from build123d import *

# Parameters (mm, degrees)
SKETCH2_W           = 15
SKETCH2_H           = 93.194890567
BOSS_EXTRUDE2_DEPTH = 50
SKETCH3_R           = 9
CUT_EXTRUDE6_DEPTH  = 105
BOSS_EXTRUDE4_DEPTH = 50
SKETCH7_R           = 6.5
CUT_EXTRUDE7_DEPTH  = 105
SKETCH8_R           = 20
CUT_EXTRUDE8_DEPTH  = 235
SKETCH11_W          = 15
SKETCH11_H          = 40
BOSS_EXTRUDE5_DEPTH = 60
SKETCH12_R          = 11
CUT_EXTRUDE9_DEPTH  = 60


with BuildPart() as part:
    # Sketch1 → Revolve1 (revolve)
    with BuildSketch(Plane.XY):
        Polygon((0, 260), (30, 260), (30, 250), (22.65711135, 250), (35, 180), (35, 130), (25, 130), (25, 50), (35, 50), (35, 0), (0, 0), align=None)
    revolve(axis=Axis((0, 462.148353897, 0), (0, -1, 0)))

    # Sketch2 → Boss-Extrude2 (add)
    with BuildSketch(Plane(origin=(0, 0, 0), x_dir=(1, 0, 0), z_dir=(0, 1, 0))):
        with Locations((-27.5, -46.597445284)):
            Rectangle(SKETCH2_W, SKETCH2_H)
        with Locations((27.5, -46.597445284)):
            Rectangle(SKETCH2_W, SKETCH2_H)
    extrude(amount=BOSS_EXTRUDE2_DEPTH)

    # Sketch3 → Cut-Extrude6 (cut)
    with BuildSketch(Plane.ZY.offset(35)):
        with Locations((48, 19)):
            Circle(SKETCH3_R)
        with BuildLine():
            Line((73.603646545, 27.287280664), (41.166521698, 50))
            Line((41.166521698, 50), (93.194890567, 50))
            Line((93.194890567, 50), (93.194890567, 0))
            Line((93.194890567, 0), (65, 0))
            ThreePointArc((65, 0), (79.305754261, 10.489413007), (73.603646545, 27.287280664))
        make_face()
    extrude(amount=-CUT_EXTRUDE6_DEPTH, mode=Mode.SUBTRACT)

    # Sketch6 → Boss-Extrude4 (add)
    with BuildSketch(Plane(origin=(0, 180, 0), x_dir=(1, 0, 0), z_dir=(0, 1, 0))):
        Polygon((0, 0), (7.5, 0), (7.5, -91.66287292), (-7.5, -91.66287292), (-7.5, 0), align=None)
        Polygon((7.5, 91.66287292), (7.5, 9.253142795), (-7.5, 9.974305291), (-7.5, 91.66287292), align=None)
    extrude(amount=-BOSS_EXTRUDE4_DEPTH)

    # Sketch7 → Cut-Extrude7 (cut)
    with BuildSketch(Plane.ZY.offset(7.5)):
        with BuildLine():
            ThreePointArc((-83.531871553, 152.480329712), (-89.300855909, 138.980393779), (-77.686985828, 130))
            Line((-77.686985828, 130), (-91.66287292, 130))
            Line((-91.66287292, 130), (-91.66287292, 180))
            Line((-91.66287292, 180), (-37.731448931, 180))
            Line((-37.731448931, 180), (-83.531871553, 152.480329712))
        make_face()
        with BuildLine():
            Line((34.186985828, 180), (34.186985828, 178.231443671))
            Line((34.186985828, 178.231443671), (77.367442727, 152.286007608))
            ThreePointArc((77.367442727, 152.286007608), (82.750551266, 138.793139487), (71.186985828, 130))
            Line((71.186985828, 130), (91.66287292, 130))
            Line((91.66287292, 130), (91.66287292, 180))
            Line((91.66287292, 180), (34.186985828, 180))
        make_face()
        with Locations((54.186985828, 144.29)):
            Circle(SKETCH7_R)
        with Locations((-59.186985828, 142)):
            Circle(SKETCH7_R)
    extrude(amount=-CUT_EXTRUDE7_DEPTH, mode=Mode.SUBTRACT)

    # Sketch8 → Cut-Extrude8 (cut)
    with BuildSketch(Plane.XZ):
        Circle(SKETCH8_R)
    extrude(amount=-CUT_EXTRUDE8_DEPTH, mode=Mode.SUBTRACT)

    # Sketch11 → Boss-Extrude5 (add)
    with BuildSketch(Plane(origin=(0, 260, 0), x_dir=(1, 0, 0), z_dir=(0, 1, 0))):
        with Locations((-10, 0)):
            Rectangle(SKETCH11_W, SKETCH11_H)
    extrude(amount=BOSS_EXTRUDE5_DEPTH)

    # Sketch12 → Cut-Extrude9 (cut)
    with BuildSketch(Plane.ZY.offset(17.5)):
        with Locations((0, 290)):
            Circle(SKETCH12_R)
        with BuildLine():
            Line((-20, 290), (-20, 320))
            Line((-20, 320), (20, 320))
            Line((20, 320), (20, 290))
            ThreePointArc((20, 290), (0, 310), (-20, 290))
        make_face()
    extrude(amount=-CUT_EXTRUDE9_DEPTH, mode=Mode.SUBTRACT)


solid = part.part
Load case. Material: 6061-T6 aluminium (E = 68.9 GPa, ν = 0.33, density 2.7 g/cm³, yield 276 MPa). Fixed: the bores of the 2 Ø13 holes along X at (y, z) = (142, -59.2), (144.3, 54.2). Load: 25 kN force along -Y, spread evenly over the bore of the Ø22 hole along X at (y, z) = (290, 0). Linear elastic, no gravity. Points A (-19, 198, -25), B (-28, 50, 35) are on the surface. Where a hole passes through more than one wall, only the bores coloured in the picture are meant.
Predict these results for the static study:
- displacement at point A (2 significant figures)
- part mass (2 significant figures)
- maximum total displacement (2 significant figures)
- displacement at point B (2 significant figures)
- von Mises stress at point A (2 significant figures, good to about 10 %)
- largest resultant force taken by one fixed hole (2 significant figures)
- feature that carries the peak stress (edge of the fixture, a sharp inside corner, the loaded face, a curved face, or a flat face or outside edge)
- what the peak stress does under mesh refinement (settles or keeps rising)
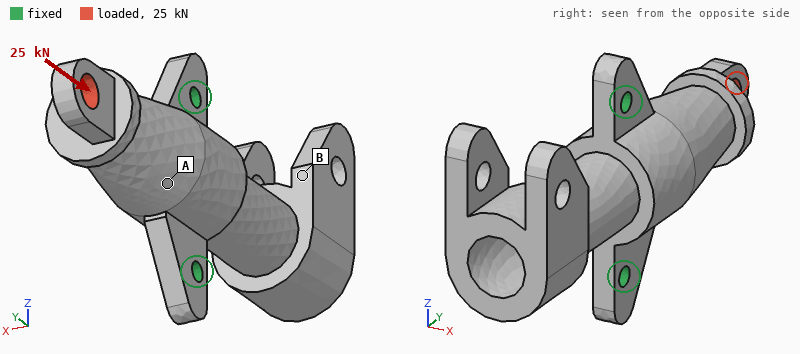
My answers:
0.17 mm
1.6 kg
0.52 mm
0.27 mm
22 MPa
14 kN
edge of the fixture
keeps rising
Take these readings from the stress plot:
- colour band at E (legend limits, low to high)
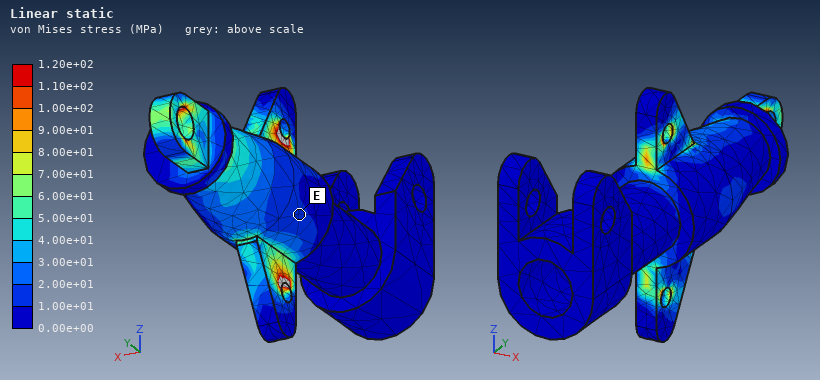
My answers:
1.00e+01 to 2.00e+01 MPa
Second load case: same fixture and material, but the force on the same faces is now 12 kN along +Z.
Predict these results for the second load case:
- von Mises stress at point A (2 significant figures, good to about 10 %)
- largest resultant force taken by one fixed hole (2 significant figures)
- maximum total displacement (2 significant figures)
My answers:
44 MPa
18 kN
0.55 mm
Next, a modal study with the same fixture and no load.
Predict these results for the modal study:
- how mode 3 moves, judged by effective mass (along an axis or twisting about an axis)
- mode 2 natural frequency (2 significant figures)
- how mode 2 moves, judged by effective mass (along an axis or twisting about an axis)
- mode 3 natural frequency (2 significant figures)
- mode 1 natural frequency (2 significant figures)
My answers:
along X
840 Hz
along Z
1400 Hz
410 Hz
